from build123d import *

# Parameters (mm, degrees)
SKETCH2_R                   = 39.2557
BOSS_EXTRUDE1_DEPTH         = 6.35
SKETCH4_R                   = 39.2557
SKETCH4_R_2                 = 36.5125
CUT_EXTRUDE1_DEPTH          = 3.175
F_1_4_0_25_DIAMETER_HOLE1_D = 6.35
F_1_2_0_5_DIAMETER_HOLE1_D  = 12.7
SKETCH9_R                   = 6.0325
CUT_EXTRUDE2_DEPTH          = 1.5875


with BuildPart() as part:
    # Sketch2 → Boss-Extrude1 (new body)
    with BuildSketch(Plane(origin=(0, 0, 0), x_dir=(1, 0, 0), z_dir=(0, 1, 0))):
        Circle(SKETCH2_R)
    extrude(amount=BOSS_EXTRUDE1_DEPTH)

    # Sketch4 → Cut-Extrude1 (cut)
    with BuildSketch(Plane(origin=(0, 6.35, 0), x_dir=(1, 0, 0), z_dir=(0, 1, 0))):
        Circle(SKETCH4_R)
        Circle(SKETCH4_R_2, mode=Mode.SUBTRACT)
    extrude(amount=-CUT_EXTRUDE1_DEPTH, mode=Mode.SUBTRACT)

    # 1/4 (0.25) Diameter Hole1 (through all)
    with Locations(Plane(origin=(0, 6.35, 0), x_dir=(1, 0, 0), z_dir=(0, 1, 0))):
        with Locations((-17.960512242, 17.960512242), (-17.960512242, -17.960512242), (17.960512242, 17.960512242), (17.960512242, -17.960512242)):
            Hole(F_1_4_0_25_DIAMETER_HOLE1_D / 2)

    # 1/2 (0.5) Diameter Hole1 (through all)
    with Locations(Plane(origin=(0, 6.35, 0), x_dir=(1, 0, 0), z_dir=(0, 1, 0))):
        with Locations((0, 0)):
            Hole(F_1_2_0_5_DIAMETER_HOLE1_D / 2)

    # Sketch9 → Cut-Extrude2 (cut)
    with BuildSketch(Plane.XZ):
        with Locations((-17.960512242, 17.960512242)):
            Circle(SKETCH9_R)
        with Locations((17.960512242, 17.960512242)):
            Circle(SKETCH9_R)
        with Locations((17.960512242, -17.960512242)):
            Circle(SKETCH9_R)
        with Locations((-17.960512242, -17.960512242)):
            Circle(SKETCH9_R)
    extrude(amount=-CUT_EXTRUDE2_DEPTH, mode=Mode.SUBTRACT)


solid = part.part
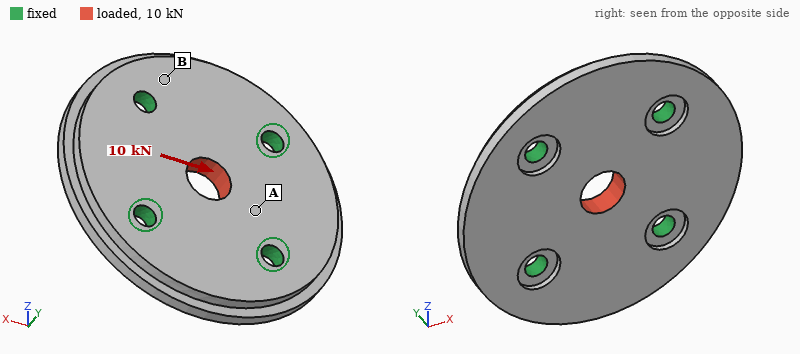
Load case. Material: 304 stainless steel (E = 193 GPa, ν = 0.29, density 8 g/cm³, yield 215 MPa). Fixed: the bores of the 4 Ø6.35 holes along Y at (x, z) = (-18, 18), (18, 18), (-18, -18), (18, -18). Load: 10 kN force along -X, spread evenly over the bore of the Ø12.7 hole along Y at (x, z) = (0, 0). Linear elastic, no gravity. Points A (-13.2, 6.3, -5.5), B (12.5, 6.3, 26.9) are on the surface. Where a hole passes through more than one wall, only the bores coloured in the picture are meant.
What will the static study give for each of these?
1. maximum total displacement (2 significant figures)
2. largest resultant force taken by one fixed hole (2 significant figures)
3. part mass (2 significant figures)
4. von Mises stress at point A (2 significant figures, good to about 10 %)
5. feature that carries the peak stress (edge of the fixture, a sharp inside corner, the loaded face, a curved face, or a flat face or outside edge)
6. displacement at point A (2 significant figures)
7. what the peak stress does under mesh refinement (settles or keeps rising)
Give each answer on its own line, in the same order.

4.1 µm
2.6 kN
210 g
26 MPa
edge of the fixture
2.3 µm
keeps rising
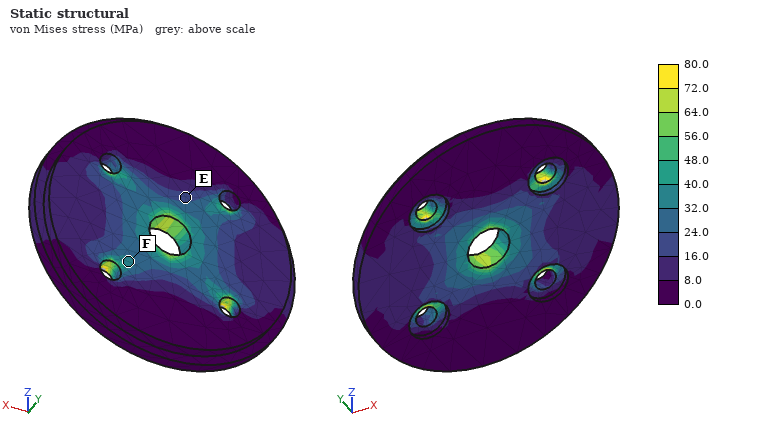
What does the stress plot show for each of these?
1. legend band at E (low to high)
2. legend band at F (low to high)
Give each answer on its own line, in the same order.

16.0 to 24.0 MPa
32.0 to 40.0 MPa
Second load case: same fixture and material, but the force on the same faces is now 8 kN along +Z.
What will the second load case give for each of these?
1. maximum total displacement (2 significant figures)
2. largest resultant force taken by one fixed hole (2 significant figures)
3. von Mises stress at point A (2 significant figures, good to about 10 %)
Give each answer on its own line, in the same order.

3.3 µm
2.1 kN
19 MPa
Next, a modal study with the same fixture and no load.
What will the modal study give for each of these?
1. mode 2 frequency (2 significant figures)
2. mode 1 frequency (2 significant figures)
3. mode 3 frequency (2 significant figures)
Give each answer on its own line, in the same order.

11 kHz
10 kHz
11 kHz
